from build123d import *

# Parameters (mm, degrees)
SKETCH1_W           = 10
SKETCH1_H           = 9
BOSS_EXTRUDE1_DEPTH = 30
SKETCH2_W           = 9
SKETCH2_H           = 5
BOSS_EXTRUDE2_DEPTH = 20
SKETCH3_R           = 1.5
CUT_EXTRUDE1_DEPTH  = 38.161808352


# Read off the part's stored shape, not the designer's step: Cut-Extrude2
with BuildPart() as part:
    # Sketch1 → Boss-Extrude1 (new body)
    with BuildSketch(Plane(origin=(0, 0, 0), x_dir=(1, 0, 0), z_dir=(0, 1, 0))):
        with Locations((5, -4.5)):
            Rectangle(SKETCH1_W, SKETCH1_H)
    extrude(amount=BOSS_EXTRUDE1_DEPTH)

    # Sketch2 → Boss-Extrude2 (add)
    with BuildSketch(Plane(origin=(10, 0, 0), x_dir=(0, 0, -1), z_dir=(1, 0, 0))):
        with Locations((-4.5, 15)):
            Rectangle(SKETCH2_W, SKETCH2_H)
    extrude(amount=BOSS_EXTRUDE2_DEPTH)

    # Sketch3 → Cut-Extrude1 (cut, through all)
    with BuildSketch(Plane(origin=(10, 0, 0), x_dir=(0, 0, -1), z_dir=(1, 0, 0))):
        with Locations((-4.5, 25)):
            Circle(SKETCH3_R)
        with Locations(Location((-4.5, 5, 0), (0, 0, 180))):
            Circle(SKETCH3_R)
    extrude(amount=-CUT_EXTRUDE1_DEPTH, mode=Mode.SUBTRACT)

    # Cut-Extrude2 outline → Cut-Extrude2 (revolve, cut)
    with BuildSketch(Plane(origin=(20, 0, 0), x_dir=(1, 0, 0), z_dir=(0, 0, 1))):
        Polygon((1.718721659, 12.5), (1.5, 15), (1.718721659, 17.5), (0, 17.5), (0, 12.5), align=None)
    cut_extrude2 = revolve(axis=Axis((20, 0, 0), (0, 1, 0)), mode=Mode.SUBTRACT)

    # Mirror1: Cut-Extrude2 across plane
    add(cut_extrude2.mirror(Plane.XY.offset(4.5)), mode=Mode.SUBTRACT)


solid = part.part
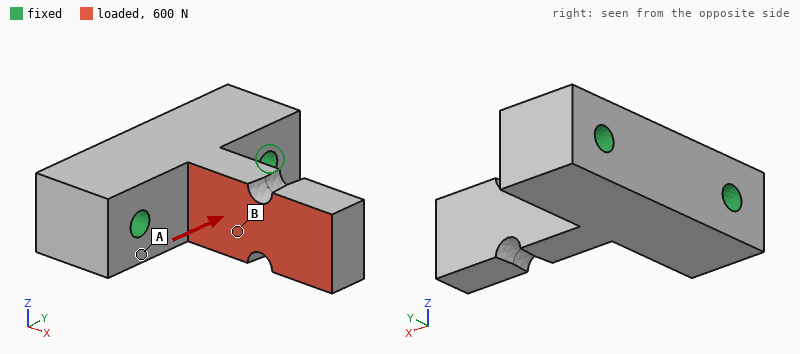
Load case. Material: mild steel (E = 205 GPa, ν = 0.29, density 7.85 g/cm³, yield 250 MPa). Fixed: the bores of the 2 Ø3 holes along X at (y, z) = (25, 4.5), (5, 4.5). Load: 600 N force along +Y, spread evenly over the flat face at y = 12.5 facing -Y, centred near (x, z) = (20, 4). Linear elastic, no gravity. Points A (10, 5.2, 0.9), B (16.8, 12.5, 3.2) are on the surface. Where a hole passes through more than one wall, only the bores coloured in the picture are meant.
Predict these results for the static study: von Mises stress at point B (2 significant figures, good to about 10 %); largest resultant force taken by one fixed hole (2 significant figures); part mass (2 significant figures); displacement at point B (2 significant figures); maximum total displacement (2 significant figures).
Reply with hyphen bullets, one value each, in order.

- 86 MPa
- 600 N
- 27 g
- 13 µm
- 49 µm
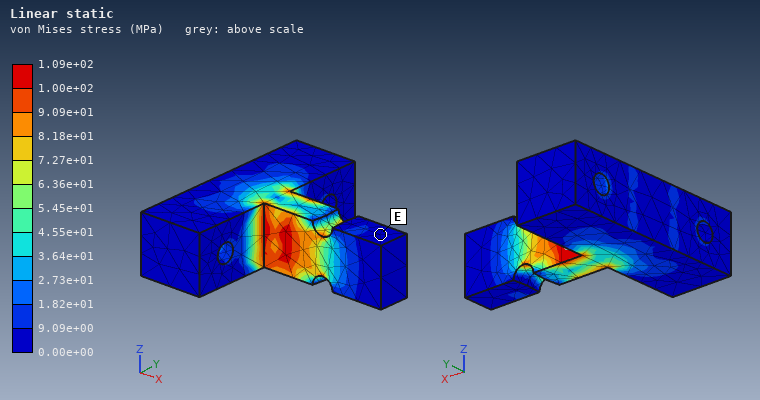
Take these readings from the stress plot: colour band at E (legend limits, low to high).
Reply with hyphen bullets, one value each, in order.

- 0.00e+00 to 9.09e+00 MPa
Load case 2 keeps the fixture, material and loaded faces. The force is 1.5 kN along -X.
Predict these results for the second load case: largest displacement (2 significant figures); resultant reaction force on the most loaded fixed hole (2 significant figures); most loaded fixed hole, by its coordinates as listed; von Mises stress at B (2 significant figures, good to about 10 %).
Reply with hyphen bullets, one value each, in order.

- 37 µm
- 1000 N
- (5, 4.5)
- 100 MPa
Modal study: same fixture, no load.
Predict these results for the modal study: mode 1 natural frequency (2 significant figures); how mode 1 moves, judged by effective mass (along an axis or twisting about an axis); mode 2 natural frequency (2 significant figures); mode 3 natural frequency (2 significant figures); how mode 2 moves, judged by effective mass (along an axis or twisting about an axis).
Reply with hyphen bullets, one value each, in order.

- 8300 Hz
- along Y
- 10 kHz
- 30 kHz
- along Z
